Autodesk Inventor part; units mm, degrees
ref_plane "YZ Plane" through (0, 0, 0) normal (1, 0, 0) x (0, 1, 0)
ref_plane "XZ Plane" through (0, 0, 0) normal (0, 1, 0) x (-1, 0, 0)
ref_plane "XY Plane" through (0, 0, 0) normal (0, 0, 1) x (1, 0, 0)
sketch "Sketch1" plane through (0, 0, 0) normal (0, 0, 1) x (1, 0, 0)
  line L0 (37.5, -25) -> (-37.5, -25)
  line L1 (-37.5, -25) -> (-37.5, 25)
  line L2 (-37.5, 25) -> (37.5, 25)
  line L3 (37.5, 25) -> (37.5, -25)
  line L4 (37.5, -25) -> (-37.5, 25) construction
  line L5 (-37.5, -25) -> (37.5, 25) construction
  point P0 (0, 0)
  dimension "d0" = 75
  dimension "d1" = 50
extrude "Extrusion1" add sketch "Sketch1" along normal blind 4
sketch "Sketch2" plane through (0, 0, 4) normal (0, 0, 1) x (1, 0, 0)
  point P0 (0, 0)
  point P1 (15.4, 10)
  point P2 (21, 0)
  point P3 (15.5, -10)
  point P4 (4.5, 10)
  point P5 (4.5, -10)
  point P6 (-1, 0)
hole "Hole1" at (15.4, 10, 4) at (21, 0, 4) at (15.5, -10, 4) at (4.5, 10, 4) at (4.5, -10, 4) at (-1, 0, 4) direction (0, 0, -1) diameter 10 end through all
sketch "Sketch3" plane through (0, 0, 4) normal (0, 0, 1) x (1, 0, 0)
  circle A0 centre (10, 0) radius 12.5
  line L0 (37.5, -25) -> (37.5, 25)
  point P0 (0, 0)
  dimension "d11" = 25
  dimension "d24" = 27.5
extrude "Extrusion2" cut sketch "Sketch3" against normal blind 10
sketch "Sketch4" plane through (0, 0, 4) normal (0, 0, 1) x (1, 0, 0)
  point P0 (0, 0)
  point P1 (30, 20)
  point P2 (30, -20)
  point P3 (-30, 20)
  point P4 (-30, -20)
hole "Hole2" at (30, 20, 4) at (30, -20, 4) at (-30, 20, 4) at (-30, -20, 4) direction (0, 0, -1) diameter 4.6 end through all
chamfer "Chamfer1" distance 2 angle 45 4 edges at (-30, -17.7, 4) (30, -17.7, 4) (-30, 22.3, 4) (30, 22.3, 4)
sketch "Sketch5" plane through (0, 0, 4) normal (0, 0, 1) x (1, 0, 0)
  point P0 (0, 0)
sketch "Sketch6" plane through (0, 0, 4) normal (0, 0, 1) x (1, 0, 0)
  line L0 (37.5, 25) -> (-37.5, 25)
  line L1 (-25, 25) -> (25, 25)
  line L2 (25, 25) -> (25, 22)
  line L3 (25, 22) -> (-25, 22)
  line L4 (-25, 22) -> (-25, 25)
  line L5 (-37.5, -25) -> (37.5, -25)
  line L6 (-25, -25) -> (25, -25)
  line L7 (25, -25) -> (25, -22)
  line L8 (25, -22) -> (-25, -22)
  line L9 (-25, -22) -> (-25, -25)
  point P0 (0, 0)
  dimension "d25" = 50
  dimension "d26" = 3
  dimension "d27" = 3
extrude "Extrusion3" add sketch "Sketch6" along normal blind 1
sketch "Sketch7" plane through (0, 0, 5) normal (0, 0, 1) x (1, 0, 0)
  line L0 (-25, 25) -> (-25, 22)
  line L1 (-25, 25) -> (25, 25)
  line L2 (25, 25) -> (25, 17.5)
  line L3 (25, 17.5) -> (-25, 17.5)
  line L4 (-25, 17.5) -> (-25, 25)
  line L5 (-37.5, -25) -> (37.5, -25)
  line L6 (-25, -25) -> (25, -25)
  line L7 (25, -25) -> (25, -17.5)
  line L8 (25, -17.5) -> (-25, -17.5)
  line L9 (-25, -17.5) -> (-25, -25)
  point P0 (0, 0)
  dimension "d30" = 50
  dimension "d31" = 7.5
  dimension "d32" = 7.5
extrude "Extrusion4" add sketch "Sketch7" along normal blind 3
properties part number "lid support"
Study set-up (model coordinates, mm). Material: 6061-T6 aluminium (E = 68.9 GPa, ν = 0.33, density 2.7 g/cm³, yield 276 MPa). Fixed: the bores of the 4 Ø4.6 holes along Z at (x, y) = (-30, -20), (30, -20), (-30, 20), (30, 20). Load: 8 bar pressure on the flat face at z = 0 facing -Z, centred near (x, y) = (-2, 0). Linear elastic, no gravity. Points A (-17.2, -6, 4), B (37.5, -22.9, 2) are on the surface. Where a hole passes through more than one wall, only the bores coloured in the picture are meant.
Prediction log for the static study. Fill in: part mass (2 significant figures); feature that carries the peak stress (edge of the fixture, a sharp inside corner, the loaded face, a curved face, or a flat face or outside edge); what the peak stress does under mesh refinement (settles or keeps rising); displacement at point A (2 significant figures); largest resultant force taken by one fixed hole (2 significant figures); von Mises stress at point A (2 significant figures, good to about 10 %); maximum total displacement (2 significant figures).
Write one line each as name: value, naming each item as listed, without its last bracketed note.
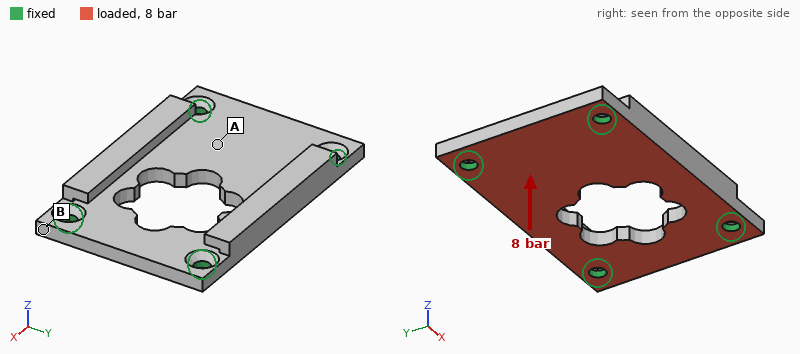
part mass: 39 g
feature that carries the peak stress: edge of the fixture
what the peak stress does under mesh refinement: keeps rising
displacement at point A: 55 µm
largest resultant force taken by one fixed hole: 810 N
von Mises stress at point A: 27 MPa
maximum total displacement: 93 µm
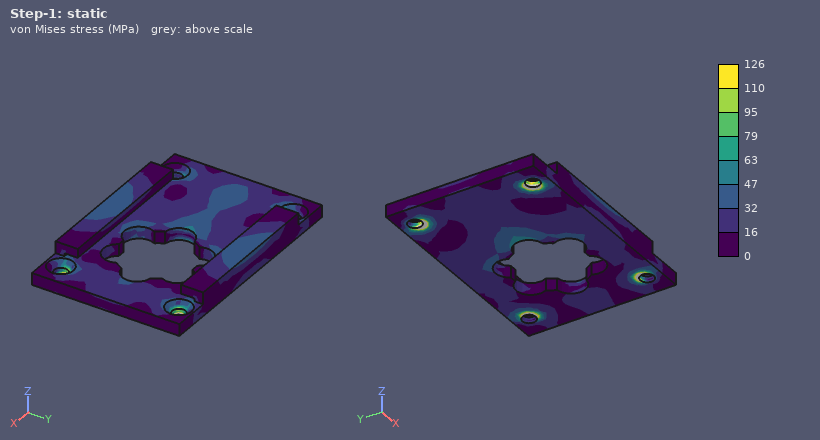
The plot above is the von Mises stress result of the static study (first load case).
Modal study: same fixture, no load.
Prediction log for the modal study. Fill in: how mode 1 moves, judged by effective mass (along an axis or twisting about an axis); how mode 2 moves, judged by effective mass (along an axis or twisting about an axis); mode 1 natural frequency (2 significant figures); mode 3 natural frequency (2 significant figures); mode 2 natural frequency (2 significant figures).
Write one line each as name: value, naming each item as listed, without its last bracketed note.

how mode 1 moves, judged by effective mass: along Z
how mode 2 moves, judged by effective mass: twisting about X
mode 1 natural frequency: 5600 Hz
mode 3 natural frequency: 9500 Hz
mode 2 natural frequency: 7800 Hz
